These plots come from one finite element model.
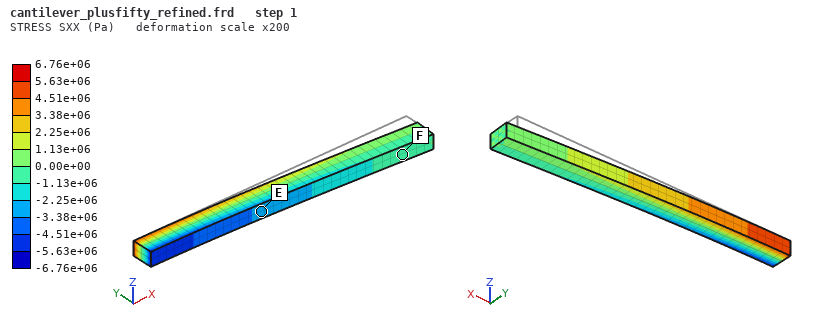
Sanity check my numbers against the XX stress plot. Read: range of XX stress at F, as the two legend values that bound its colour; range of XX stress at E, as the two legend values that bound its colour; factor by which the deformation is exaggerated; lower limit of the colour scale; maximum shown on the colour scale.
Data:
-1.13e+06 to 0.00e+00 Pa
-3.38e+06 to -2.25e+06 Pa
200
-6.76e+06 Pa
6.76e+06 Pa
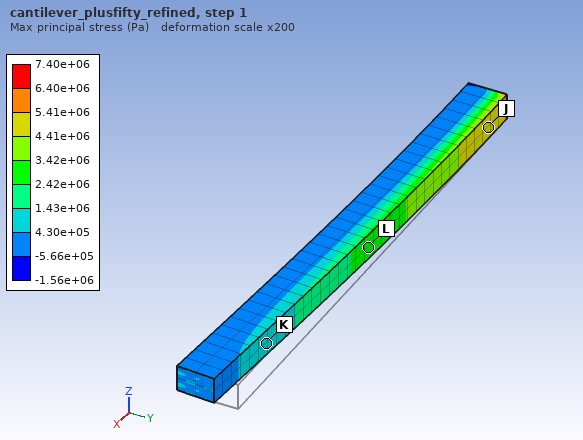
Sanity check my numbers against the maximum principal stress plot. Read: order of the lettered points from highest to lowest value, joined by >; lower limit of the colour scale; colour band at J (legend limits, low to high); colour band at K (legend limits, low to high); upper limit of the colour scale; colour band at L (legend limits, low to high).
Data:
J > L > K
-1.56e+06 Pa
4.41e+06 to 5.41e+06 Pa
4.30e+05 to 1.43e+06 Pa
7.40e+06 Pa
2.42e+06 to 3.42e+06 Pa
